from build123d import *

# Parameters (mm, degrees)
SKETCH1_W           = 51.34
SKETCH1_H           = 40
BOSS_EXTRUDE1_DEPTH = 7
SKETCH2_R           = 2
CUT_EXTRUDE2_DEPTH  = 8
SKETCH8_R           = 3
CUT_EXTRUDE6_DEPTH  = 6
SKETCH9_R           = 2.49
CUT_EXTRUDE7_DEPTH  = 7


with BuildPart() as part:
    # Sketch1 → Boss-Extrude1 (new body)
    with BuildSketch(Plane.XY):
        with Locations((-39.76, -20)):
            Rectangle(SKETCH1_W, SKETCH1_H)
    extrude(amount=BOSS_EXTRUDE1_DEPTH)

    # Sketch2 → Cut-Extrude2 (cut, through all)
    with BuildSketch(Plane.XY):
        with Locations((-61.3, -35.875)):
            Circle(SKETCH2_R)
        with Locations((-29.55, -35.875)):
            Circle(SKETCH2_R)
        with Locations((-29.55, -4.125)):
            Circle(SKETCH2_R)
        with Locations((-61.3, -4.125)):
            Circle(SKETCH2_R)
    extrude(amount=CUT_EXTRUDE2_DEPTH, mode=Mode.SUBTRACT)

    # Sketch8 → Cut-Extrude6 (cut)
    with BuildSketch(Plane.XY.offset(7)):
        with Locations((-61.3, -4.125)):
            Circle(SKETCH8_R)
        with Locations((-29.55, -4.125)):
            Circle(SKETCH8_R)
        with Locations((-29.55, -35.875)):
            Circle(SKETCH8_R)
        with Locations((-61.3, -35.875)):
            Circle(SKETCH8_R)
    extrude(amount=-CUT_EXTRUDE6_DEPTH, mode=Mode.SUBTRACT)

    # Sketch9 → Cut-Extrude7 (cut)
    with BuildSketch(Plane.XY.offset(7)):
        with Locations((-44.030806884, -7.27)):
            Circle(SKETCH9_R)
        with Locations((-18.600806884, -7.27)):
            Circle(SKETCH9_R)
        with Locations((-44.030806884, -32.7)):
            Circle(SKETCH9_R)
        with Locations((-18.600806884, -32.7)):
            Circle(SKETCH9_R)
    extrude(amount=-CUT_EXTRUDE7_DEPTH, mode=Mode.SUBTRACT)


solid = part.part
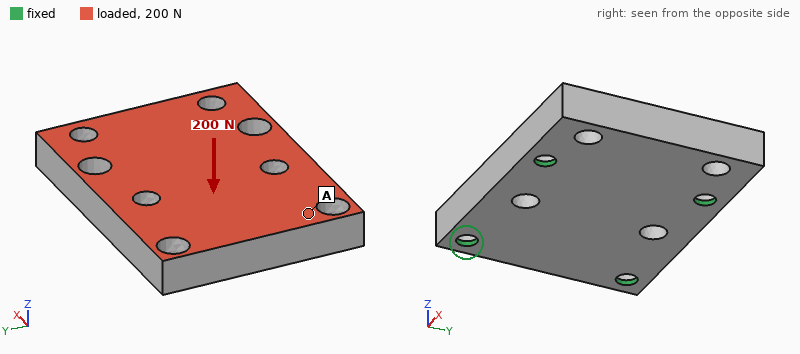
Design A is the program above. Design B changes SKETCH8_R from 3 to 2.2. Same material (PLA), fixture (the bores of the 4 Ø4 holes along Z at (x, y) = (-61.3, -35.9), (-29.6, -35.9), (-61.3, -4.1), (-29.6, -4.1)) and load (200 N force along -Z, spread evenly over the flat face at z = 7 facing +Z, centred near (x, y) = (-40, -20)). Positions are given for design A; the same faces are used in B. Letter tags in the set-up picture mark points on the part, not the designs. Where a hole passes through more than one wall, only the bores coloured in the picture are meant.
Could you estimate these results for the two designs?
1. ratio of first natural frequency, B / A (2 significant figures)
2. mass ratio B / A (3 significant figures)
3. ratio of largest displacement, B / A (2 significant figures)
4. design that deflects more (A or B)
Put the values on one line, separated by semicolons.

1.1; 1.02; 0.76; A
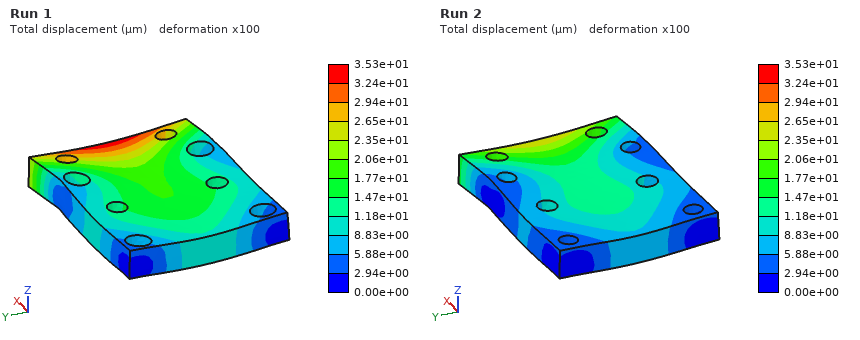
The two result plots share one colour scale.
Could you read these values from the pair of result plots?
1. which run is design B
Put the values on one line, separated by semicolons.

Run 2
